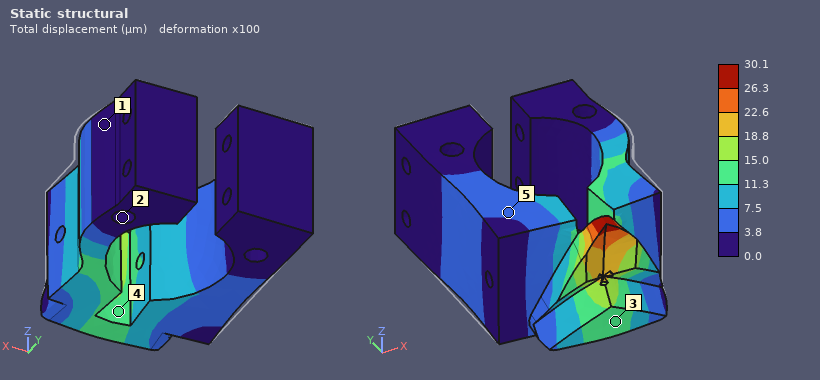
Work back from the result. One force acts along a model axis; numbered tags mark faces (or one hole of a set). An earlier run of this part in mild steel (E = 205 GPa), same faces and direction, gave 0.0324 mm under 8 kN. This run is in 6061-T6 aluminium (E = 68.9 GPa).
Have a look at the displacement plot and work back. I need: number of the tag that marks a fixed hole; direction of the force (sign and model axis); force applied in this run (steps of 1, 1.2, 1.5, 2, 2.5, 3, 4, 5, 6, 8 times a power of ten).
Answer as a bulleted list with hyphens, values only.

- 2
- -Y
- 2.5 kN
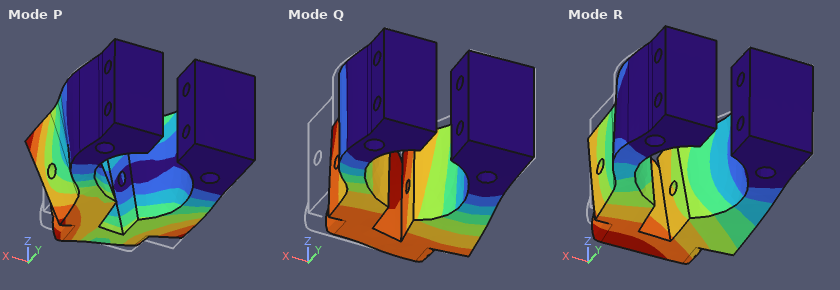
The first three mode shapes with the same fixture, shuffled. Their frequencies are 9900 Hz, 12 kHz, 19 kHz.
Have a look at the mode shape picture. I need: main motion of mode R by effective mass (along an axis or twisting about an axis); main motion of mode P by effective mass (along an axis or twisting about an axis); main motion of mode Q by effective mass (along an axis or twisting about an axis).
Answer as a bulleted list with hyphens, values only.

- along Z
- twisting about Y
- along X
